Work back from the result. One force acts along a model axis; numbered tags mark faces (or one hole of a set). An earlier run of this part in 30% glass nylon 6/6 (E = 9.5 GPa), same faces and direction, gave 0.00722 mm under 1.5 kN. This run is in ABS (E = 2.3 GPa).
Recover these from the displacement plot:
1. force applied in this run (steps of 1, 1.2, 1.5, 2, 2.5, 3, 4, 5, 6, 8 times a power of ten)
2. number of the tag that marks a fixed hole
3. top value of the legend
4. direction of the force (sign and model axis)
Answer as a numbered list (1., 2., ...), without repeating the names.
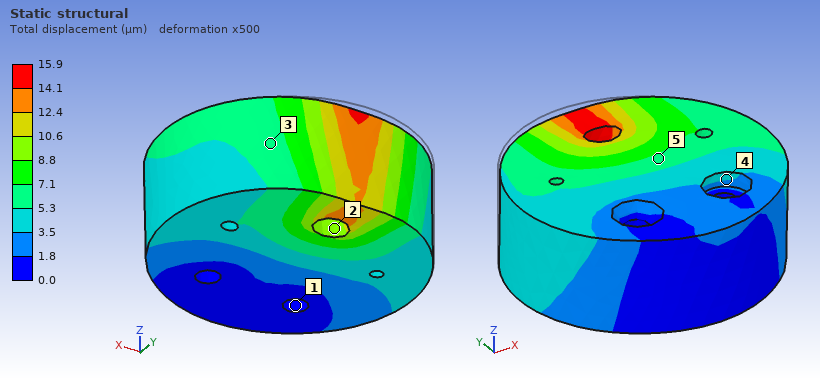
1. 800 N
2. 1
3. 15.9 µm
4. -Y
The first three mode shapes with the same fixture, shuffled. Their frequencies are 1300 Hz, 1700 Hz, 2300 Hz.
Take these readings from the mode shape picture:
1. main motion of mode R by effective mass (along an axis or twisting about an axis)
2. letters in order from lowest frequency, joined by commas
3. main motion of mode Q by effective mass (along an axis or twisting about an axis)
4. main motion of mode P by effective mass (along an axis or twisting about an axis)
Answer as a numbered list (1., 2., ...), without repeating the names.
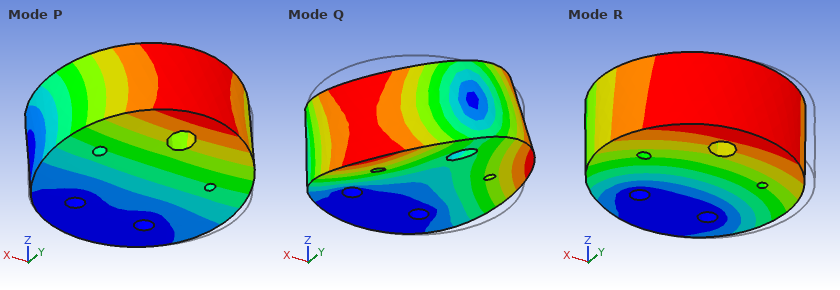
1. along X
2. P, R, Q
3. twisting about Y
4. along Z
